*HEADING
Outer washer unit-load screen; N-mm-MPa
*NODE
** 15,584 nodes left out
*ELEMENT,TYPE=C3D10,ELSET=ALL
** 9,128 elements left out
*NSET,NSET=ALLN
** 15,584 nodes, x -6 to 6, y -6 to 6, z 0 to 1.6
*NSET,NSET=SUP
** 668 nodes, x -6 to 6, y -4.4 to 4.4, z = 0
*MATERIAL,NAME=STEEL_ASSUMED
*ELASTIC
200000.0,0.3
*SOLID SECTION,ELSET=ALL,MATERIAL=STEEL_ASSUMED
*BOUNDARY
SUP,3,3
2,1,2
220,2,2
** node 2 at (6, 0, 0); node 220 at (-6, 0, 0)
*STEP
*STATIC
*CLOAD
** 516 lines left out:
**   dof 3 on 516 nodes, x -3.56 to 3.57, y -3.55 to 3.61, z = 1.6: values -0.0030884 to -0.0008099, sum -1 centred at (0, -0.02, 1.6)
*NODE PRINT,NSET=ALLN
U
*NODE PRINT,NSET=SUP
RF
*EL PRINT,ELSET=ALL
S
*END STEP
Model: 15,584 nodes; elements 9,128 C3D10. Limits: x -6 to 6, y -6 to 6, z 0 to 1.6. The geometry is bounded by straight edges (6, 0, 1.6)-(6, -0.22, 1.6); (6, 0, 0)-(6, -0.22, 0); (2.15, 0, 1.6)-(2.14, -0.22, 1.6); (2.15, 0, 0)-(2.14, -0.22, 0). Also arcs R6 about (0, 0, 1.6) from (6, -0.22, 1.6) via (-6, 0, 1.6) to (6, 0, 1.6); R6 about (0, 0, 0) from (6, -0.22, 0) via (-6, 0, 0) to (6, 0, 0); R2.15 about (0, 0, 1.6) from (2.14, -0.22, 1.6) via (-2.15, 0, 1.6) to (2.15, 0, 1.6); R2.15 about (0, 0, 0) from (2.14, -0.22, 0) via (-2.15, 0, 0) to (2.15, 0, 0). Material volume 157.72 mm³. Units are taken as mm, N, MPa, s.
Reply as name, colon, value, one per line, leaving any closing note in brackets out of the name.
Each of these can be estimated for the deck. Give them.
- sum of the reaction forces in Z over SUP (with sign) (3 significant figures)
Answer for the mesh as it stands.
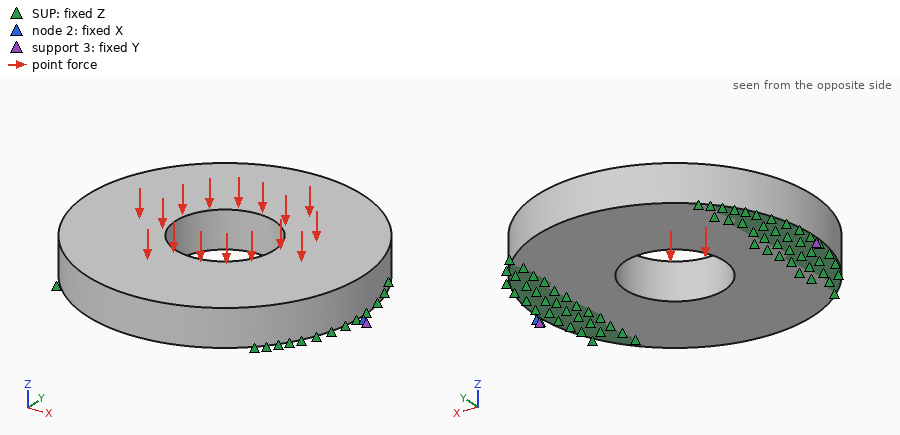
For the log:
sum of the reaction forces in Z over SUP (with sign): 1.00 N
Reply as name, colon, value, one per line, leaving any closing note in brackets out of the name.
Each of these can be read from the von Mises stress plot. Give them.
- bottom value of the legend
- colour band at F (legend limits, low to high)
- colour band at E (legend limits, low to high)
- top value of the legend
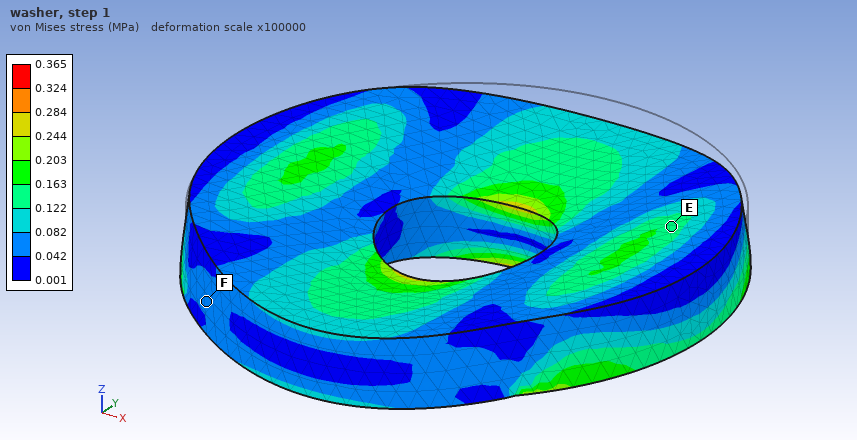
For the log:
bottom value of the legend: 0.001 MPa
colour band at F: 0.042 to 0.082 MPa
colour band at E: 0.122 to 0.163 MPa
top value of the legend: 0.365 MPa
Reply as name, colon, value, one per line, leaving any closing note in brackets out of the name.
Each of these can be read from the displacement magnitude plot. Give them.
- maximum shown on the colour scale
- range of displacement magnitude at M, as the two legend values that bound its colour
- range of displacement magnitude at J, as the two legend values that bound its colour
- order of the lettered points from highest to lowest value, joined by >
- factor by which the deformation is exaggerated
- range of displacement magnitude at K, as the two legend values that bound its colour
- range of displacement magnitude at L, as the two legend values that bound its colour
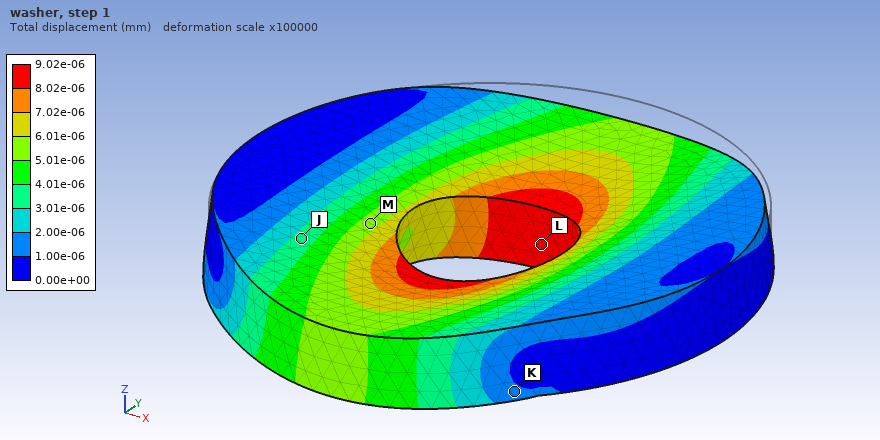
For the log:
maximum shown on the colour scale: 9.02e-06 mm
range of displacement magnitude at M, as the two legend values that bound its colour: 5.01e-06 to 6.01e-06 mm
range of displacement magnitude at J, as the two legend values that bound its colour: 3.01e-06 to 4.01e-06 mm
order of the lettered points from highest to lowest value, joined by >: L > M > J > K
factor by which the deformation is exaggerated: 100000
range of displacement magnitude at K, as the two legend values that bound its colour: 1.00e-06 to 2.00e-06 mm
range of displacement magnitude at L, as the two legend values that bound its colour: 8.02e-06 to 9.02e-06 mm
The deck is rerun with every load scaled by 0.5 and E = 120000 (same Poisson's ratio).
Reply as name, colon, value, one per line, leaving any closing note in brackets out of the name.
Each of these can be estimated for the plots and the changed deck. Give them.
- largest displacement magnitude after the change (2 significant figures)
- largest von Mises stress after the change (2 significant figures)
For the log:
largest displacement magnitude after the change: 7.5e-06 mm
largest von Mises stress after the change: 0.18 MPa
